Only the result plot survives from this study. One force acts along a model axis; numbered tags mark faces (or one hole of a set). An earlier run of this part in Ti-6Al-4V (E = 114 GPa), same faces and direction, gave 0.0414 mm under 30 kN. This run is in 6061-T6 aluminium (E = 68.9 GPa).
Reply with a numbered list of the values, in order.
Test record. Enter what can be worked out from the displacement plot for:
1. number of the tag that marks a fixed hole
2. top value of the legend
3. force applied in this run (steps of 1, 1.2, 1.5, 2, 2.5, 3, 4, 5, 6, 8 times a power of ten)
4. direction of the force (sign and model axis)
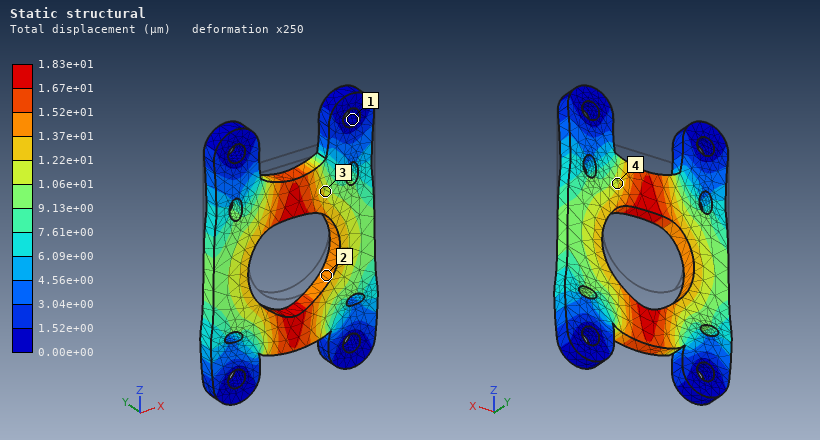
1. 1
2. 1.83e+01 µm
3. 8 kN
4. -Z
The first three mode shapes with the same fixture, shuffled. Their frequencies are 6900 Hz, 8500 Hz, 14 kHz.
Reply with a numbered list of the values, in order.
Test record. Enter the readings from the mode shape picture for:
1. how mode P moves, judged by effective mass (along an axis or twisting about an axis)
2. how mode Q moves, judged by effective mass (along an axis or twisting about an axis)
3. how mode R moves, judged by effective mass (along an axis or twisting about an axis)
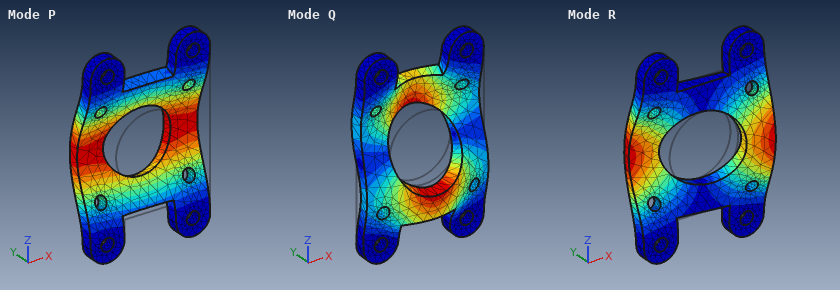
1. along Y
2. twisting about X
3. twisting about Z
